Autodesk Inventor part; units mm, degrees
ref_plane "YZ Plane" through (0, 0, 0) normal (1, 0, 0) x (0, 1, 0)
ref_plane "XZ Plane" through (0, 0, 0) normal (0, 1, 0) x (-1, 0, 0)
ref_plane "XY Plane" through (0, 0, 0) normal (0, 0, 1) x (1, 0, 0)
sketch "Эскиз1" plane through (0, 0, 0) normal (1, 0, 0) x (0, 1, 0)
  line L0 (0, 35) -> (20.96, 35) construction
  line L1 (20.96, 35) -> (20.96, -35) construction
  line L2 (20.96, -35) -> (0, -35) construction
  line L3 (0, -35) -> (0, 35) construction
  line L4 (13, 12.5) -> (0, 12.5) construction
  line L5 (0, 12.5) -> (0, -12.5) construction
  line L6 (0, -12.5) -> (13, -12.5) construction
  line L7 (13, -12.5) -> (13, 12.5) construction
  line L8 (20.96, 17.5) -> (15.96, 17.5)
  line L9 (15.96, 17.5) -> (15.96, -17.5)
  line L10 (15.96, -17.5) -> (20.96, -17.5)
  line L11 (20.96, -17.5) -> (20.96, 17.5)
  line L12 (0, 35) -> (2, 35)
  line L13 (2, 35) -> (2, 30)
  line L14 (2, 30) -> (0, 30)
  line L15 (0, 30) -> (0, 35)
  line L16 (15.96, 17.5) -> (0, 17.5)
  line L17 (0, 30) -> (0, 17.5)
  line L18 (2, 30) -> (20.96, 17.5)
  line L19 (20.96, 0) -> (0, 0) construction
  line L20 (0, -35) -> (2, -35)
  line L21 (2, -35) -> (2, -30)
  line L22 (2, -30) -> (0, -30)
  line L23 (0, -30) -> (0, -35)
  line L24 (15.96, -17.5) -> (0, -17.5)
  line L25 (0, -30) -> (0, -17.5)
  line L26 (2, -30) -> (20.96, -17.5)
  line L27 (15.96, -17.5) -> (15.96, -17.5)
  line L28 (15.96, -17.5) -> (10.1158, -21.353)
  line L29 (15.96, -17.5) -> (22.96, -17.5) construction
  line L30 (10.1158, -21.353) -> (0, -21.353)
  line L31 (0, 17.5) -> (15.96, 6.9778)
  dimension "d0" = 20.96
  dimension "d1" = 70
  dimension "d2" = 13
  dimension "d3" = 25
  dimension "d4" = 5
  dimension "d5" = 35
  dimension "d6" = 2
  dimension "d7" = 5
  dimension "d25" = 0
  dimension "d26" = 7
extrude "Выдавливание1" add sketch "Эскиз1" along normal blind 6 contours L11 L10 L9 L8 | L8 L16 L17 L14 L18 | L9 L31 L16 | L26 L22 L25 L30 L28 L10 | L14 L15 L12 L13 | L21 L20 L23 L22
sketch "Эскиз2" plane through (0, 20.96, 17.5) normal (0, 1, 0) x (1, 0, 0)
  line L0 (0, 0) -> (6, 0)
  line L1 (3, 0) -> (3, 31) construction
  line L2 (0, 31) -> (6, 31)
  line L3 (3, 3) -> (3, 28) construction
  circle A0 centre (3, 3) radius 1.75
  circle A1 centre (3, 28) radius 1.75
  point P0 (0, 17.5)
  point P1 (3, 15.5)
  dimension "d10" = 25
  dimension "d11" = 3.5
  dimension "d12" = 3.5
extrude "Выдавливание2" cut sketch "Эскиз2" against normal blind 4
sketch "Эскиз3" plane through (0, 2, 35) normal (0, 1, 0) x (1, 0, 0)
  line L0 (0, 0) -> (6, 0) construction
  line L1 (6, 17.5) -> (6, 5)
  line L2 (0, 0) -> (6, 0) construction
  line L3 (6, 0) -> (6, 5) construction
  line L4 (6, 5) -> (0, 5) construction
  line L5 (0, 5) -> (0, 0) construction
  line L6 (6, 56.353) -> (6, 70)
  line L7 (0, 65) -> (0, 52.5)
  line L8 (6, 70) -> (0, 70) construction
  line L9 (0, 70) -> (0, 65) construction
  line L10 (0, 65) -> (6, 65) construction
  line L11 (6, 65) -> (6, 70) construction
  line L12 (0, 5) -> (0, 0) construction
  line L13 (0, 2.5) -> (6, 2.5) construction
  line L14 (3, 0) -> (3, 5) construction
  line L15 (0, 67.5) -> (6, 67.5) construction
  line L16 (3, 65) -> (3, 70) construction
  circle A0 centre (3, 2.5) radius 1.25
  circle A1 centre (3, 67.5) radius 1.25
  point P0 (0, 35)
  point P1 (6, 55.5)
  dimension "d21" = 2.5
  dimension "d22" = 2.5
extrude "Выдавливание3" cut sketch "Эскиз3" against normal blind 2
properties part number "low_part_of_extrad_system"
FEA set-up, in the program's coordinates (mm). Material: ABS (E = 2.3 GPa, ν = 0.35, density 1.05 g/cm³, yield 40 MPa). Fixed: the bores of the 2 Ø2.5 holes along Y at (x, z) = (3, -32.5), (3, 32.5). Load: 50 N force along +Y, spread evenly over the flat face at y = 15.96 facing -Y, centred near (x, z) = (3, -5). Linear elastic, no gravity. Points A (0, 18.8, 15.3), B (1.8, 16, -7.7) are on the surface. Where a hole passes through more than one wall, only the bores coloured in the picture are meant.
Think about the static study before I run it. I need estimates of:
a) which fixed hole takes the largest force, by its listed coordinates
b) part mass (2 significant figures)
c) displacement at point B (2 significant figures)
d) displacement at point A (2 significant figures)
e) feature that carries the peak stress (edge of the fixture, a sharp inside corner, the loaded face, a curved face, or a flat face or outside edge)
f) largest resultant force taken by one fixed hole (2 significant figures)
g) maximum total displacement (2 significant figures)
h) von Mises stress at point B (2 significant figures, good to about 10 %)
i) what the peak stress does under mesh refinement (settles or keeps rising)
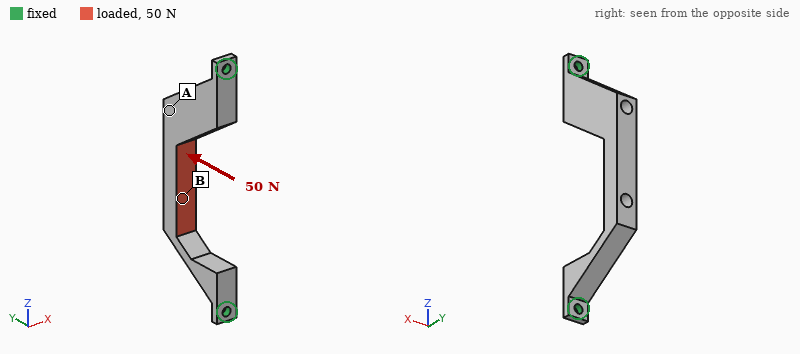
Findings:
(3, -32.5)
3.1 g
0.13 mm
0.097 mm
edge of the fixture
39 N
0.14 mm
3.5 MPa
keeps rising
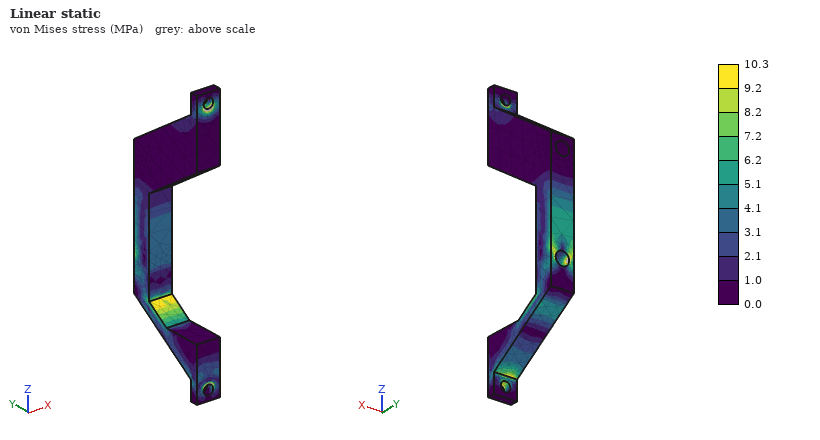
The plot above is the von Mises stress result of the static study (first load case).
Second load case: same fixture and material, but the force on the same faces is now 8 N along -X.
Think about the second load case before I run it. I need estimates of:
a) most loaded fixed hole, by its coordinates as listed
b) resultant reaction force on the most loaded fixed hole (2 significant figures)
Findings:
(3, -32.5)
4.7 N
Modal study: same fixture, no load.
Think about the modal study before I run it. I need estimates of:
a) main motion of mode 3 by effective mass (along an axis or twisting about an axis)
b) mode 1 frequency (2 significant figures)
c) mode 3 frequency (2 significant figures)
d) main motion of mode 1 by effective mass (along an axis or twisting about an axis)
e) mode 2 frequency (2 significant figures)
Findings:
twisting about Y
660 Hz
2100 Hz
along X
1700 Hz
